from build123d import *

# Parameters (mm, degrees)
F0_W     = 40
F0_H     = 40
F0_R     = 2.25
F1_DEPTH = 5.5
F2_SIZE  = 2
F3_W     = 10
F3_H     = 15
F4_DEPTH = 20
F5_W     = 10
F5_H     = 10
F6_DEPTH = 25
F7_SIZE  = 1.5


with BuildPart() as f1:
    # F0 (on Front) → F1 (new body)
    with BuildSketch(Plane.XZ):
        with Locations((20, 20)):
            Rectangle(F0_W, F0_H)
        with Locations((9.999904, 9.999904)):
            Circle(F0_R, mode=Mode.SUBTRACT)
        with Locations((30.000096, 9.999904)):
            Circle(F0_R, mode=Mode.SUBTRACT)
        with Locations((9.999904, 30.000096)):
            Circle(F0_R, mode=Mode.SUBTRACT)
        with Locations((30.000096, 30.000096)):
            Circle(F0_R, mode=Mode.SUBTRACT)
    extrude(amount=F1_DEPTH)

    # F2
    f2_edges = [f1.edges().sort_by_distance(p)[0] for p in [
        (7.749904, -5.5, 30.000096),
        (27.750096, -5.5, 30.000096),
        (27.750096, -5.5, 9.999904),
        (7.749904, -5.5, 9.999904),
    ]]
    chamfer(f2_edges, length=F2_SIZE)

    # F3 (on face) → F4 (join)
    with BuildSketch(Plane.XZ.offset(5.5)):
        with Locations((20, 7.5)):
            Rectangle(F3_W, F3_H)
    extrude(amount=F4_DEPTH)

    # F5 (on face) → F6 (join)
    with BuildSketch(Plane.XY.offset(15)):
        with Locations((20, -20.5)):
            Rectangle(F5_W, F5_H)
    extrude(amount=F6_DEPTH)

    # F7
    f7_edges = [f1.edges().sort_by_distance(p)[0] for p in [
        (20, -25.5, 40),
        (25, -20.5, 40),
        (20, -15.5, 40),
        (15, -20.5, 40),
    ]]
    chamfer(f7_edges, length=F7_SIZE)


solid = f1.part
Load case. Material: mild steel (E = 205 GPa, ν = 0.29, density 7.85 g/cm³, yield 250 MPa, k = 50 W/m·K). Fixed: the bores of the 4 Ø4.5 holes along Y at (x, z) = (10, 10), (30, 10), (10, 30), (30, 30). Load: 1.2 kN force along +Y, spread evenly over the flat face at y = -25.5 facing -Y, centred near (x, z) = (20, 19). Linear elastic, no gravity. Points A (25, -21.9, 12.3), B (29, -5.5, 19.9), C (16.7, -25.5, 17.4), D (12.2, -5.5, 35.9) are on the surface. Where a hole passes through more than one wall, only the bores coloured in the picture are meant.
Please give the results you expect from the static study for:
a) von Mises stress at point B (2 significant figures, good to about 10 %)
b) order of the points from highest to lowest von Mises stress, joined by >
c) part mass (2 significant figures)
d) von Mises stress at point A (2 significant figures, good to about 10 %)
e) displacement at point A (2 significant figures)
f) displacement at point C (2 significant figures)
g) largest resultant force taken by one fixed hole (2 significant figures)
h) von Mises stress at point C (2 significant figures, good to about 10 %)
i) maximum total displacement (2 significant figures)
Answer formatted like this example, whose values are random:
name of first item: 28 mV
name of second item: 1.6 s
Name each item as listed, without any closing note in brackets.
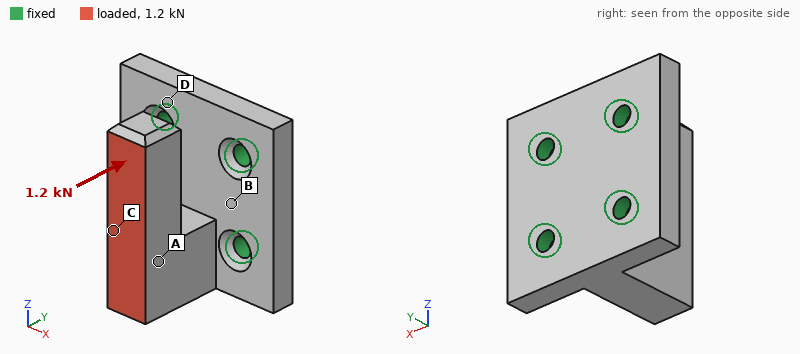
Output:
von Mises stress at point B: 14 MPa
order of the points from highest to lowest von Mises stress, joined by >: C > A > B > D
part mass: 110 g
von Mises stress at point A: 23 MPa
displacement at point A: 12 µm
displacement at point C: 18 µm
largest resultant force taken by one fixed hole: 480 N
von Mises stress at point C: 43 MPa
maximum total displacement: 42 µm
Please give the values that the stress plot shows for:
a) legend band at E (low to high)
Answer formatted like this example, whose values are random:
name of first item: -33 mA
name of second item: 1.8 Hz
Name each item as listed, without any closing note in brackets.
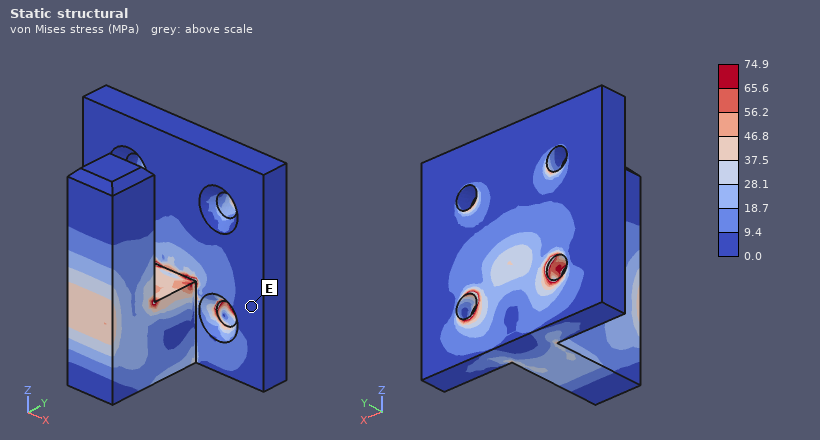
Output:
legend band at E: 0.0 to 9.4 MPa
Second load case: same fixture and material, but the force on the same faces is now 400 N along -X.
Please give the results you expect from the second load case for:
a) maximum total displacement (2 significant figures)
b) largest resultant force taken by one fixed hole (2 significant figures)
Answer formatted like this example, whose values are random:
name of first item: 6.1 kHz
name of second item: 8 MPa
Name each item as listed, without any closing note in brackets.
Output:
maximum total displacement: 23 µm
largest resultant force taken by one fixed hole: 570 N
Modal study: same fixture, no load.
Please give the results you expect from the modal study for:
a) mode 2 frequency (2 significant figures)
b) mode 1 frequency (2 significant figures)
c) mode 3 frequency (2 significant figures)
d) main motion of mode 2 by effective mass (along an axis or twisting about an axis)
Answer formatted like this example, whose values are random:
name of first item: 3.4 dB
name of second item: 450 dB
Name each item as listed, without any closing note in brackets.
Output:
mode 2 frequency: 5000 Hz
mode 1 frequency: 4700 Hz
mode 3 frequency: 11 kHz
main motion of mode 2 by effective mass: along X
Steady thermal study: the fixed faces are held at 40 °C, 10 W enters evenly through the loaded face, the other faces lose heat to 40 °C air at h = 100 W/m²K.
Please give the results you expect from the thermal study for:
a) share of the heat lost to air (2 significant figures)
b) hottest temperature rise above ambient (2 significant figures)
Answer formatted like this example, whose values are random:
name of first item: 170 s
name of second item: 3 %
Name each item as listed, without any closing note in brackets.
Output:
share of the heat lost to air: 39 %
hottest temperature rise above ambient: 31 K
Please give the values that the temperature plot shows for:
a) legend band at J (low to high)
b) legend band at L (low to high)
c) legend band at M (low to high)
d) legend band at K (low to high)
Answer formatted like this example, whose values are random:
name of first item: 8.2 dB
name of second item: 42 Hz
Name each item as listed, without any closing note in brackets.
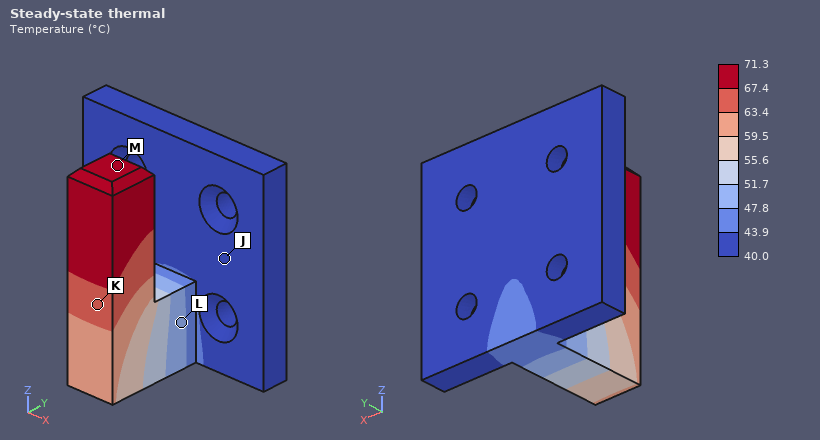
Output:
legend band at J: 40.0 to 43.9 °C
legend band at L: 47.8 to 51.7 °C
legend band at M: 67.4 to 71.3 °C
legend band at K: 63.4 to 67.4 °C
